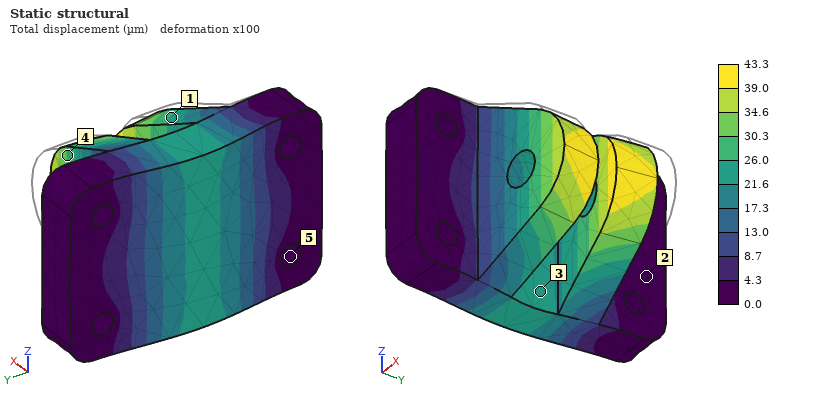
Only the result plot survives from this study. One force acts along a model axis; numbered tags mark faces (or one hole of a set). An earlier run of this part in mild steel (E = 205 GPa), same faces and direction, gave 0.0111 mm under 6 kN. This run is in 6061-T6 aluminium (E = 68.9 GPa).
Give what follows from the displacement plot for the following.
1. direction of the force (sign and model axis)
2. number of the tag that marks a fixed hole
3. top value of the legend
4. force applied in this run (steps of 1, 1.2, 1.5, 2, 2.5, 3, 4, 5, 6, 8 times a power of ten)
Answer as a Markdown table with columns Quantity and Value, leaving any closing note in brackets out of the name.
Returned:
| Quantity | Value |
|---|---|
| direction of the force | -X |
| number of the tag that marks a fixed hole | 5 |
| top value of the legend | 43.3 µm |
| force applied in this run | 8 kN |
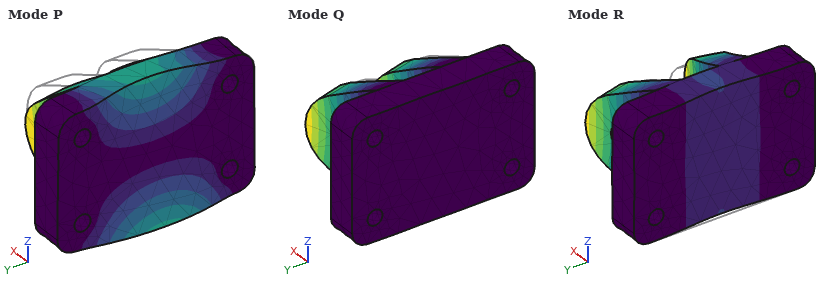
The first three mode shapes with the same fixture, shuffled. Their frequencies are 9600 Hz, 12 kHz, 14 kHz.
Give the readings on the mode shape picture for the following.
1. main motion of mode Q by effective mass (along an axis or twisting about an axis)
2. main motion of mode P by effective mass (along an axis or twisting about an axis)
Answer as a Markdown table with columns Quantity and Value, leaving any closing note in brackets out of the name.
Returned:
| Quantity | Value |
|---|---|
| main motion of mode Q by effective mass | along Y |
| main motion of mode P by effective mass | along Z |
